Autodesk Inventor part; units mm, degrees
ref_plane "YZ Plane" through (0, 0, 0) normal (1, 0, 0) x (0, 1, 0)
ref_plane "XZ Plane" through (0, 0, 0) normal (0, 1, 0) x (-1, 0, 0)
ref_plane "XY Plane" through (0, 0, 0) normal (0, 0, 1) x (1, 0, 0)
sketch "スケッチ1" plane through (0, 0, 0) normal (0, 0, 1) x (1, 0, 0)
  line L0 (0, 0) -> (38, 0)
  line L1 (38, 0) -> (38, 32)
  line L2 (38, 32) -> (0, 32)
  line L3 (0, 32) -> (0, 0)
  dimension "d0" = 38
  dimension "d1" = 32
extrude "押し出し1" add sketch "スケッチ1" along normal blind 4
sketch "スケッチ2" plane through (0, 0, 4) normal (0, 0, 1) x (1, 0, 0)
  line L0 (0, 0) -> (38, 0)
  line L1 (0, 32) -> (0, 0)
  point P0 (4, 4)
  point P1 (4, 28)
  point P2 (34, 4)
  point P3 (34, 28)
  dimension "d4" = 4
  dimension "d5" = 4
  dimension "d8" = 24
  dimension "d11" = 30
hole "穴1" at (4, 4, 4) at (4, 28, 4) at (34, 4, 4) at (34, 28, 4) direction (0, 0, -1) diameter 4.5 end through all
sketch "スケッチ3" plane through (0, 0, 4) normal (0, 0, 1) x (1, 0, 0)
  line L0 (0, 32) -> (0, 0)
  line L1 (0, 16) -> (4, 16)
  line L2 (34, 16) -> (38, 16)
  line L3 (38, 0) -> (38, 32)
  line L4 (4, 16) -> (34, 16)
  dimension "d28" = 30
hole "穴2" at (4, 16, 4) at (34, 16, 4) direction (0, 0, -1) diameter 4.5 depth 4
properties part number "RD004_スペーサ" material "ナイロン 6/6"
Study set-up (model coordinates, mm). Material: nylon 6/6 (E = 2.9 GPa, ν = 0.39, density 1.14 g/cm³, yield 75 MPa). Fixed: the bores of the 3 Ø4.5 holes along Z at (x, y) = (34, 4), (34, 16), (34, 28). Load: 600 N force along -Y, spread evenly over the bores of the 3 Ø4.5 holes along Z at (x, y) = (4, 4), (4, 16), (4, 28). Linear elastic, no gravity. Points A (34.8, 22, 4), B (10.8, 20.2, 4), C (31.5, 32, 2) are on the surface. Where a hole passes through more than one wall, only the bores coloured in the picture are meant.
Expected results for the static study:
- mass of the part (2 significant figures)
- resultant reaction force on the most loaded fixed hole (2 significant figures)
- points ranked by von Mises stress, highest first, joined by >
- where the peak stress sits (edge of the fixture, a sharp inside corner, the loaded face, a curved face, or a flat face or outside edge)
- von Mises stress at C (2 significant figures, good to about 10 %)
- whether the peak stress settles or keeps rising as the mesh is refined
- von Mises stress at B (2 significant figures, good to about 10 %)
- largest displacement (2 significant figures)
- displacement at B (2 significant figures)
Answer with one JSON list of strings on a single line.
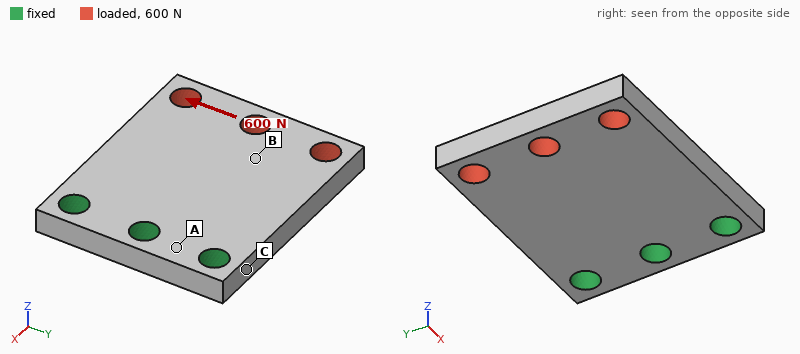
["5.1 g", "710 N", "C > B > A", "edge of the fixture", "21 MPa", "keeps rising", "10 MPa", "0.39 mm", "0.21 mm"]
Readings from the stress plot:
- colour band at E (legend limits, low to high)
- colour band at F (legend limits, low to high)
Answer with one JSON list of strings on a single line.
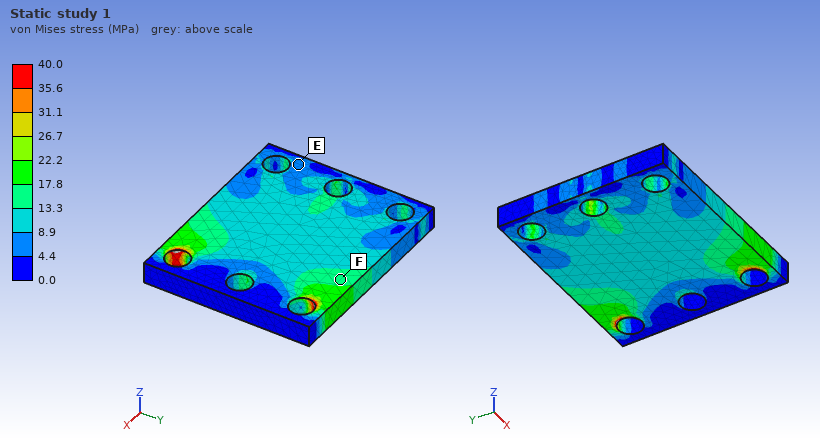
["4.4 to 8.9 MPa", "13.3 to 17.8 MPa"]
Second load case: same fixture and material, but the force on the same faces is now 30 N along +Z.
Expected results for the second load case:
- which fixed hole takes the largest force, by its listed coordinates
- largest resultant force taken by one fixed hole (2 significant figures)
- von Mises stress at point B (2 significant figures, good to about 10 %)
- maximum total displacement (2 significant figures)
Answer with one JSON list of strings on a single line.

["(34, 16)", "21 N", "2.3 MPa", "0.56 mm"]
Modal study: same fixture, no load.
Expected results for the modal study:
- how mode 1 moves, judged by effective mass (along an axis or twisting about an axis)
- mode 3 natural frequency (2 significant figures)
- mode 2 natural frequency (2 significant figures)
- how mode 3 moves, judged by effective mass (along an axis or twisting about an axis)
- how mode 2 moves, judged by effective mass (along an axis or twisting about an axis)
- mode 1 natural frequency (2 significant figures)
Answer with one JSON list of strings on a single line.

["along Z", "5200 Hz", "2400 Hz", "along Y", "twisting about X", "1100 Hz"]
